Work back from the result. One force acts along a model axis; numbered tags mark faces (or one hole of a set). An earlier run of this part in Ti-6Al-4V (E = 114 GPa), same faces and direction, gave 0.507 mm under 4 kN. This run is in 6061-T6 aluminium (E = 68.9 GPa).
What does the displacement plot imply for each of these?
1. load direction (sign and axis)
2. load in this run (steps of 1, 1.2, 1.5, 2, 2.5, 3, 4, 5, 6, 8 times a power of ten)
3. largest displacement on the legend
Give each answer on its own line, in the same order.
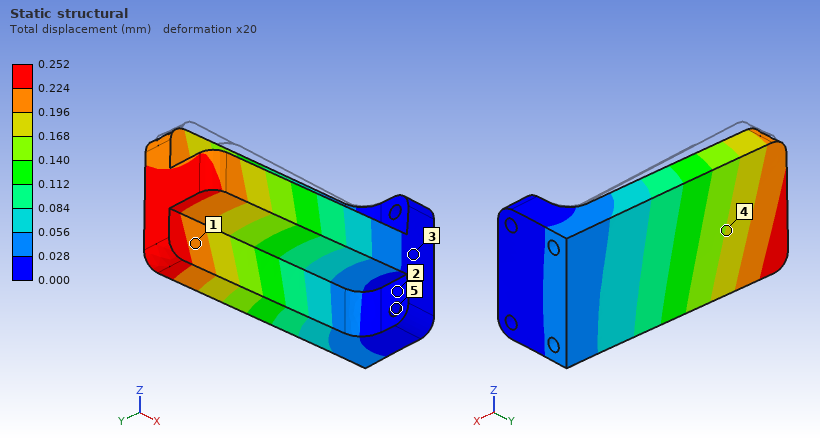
+Y
1.2 kN
0.252 mm
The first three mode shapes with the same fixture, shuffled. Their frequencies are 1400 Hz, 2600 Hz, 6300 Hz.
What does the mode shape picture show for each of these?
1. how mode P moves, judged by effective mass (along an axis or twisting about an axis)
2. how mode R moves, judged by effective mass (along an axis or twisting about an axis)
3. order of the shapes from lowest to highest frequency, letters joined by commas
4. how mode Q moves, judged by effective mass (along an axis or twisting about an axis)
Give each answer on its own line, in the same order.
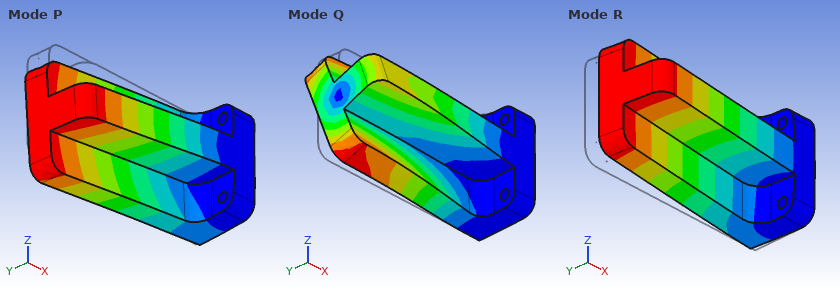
along Z
along Y
R, P, Q
twisting about X
